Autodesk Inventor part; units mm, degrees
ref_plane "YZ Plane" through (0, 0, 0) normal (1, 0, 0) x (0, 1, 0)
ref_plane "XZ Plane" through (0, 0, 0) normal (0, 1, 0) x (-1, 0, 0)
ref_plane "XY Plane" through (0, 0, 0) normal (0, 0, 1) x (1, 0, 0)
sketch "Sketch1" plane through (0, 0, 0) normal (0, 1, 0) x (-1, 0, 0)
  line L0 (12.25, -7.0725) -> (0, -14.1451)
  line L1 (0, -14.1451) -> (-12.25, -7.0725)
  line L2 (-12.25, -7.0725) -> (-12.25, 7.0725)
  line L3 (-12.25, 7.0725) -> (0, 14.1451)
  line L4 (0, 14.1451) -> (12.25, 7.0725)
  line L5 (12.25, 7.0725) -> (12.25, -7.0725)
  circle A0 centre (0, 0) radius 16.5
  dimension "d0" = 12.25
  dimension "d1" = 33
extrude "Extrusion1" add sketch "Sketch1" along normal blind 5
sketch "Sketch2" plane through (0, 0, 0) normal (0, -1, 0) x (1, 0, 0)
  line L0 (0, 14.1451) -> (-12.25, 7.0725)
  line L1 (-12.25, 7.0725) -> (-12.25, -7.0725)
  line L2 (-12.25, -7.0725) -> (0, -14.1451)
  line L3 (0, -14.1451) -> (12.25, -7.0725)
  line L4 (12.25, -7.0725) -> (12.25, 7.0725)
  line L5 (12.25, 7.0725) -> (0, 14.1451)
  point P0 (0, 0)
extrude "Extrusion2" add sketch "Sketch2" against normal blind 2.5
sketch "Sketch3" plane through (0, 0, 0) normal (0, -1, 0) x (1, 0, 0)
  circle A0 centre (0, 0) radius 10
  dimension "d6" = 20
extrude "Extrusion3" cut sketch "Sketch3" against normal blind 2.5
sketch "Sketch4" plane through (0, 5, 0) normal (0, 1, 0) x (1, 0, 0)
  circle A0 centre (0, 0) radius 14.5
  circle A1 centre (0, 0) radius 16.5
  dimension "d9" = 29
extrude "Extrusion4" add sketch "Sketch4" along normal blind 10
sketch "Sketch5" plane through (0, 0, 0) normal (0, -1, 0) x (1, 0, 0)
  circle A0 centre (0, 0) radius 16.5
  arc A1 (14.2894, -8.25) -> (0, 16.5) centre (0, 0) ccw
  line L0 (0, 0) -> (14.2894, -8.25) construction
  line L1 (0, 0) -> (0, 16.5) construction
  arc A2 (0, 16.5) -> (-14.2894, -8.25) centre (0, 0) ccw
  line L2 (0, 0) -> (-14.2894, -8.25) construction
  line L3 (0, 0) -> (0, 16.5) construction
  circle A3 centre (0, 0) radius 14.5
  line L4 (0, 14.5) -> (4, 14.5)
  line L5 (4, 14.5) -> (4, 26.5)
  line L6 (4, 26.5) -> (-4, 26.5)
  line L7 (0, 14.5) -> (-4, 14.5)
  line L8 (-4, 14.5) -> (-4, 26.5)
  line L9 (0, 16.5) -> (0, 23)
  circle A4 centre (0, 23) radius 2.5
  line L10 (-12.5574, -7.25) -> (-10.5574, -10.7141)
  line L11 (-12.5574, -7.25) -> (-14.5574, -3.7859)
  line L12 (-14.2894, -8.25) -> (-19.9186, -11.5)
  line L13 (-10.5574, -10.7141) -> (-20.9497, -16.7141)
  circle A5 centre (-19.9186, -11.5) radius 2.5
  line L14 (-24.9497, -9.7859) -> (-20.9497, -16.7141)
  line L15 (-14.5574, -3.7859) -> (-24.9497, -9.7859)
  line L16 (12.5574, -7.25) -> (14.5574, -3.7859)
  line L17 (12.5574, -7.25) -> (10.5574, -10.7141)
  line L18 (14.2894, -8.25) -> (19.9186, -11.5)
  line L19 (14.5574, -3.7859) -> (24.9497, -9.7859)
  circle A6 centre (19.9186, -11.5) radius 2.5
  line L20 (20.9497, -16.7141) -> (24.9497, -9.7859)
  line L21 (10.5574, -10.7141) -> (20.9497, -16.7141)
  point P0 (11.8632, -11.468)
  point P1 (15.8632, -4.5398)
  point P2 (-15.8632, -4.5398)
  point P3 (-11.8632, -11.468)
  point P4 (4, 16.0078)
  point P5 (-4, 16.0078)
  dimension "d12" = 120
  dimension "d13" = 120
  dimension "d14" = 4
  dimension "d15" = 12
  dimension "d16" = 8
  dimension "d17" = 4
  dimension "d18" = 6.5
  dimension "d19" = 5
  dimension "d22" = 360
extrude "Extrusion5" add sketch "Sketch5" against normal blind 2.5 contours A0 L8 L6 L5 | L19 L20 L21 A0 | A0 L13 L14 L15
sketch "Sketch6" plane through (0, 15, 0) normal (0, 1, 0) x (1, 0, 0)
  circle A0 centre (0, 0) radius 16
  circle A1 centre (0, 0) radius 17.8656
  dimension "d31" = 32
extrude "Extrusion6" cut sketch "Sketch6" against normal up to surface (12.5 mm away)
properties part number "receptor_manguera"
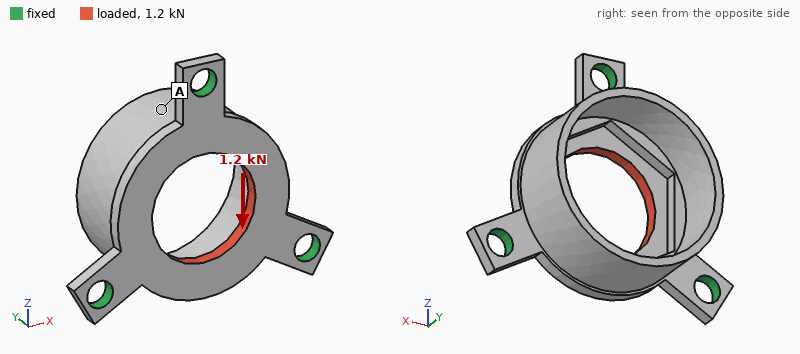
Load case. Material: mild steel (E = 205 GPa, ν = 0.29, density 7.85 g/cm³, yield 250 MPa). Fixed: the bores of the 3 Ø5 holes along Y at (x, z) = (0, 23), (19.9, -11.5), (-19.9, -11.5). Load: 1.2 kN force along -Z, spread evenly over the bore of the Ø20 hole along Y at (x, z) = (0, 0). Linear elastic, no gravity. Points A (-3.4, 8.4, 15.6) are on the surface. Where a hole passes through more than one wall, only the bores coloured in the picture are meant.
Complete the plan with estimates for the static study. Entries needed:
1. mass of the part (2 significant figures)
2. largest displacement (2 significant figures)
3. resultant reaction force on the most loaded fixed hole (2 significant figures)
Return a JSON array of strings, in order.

["31 g", "6.3 µm", "410 N"]
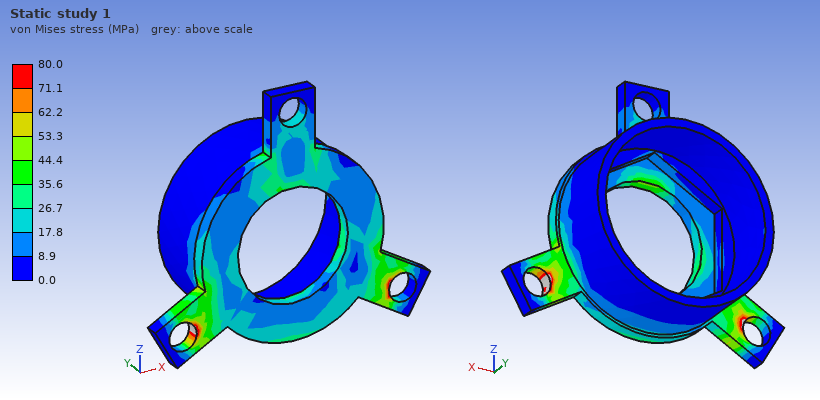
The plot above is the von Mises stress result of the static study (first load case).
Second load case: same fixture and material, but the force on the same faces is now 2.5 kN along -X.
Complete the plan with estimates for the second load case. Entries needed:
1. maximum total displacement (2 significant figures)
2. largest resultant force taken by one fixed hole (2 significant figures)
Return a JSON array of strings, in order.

["12 µm", "880 N"]
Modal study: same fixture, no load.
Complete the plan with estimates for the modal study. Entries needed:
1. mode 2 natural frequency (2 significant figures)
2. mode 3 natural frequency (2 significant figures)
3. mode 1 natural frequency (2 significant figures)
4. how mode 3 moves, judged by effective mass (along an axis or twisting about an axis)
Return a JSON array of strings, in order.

["7500 Hz", "11 kHz", "7500 Hz", "along Y"]
